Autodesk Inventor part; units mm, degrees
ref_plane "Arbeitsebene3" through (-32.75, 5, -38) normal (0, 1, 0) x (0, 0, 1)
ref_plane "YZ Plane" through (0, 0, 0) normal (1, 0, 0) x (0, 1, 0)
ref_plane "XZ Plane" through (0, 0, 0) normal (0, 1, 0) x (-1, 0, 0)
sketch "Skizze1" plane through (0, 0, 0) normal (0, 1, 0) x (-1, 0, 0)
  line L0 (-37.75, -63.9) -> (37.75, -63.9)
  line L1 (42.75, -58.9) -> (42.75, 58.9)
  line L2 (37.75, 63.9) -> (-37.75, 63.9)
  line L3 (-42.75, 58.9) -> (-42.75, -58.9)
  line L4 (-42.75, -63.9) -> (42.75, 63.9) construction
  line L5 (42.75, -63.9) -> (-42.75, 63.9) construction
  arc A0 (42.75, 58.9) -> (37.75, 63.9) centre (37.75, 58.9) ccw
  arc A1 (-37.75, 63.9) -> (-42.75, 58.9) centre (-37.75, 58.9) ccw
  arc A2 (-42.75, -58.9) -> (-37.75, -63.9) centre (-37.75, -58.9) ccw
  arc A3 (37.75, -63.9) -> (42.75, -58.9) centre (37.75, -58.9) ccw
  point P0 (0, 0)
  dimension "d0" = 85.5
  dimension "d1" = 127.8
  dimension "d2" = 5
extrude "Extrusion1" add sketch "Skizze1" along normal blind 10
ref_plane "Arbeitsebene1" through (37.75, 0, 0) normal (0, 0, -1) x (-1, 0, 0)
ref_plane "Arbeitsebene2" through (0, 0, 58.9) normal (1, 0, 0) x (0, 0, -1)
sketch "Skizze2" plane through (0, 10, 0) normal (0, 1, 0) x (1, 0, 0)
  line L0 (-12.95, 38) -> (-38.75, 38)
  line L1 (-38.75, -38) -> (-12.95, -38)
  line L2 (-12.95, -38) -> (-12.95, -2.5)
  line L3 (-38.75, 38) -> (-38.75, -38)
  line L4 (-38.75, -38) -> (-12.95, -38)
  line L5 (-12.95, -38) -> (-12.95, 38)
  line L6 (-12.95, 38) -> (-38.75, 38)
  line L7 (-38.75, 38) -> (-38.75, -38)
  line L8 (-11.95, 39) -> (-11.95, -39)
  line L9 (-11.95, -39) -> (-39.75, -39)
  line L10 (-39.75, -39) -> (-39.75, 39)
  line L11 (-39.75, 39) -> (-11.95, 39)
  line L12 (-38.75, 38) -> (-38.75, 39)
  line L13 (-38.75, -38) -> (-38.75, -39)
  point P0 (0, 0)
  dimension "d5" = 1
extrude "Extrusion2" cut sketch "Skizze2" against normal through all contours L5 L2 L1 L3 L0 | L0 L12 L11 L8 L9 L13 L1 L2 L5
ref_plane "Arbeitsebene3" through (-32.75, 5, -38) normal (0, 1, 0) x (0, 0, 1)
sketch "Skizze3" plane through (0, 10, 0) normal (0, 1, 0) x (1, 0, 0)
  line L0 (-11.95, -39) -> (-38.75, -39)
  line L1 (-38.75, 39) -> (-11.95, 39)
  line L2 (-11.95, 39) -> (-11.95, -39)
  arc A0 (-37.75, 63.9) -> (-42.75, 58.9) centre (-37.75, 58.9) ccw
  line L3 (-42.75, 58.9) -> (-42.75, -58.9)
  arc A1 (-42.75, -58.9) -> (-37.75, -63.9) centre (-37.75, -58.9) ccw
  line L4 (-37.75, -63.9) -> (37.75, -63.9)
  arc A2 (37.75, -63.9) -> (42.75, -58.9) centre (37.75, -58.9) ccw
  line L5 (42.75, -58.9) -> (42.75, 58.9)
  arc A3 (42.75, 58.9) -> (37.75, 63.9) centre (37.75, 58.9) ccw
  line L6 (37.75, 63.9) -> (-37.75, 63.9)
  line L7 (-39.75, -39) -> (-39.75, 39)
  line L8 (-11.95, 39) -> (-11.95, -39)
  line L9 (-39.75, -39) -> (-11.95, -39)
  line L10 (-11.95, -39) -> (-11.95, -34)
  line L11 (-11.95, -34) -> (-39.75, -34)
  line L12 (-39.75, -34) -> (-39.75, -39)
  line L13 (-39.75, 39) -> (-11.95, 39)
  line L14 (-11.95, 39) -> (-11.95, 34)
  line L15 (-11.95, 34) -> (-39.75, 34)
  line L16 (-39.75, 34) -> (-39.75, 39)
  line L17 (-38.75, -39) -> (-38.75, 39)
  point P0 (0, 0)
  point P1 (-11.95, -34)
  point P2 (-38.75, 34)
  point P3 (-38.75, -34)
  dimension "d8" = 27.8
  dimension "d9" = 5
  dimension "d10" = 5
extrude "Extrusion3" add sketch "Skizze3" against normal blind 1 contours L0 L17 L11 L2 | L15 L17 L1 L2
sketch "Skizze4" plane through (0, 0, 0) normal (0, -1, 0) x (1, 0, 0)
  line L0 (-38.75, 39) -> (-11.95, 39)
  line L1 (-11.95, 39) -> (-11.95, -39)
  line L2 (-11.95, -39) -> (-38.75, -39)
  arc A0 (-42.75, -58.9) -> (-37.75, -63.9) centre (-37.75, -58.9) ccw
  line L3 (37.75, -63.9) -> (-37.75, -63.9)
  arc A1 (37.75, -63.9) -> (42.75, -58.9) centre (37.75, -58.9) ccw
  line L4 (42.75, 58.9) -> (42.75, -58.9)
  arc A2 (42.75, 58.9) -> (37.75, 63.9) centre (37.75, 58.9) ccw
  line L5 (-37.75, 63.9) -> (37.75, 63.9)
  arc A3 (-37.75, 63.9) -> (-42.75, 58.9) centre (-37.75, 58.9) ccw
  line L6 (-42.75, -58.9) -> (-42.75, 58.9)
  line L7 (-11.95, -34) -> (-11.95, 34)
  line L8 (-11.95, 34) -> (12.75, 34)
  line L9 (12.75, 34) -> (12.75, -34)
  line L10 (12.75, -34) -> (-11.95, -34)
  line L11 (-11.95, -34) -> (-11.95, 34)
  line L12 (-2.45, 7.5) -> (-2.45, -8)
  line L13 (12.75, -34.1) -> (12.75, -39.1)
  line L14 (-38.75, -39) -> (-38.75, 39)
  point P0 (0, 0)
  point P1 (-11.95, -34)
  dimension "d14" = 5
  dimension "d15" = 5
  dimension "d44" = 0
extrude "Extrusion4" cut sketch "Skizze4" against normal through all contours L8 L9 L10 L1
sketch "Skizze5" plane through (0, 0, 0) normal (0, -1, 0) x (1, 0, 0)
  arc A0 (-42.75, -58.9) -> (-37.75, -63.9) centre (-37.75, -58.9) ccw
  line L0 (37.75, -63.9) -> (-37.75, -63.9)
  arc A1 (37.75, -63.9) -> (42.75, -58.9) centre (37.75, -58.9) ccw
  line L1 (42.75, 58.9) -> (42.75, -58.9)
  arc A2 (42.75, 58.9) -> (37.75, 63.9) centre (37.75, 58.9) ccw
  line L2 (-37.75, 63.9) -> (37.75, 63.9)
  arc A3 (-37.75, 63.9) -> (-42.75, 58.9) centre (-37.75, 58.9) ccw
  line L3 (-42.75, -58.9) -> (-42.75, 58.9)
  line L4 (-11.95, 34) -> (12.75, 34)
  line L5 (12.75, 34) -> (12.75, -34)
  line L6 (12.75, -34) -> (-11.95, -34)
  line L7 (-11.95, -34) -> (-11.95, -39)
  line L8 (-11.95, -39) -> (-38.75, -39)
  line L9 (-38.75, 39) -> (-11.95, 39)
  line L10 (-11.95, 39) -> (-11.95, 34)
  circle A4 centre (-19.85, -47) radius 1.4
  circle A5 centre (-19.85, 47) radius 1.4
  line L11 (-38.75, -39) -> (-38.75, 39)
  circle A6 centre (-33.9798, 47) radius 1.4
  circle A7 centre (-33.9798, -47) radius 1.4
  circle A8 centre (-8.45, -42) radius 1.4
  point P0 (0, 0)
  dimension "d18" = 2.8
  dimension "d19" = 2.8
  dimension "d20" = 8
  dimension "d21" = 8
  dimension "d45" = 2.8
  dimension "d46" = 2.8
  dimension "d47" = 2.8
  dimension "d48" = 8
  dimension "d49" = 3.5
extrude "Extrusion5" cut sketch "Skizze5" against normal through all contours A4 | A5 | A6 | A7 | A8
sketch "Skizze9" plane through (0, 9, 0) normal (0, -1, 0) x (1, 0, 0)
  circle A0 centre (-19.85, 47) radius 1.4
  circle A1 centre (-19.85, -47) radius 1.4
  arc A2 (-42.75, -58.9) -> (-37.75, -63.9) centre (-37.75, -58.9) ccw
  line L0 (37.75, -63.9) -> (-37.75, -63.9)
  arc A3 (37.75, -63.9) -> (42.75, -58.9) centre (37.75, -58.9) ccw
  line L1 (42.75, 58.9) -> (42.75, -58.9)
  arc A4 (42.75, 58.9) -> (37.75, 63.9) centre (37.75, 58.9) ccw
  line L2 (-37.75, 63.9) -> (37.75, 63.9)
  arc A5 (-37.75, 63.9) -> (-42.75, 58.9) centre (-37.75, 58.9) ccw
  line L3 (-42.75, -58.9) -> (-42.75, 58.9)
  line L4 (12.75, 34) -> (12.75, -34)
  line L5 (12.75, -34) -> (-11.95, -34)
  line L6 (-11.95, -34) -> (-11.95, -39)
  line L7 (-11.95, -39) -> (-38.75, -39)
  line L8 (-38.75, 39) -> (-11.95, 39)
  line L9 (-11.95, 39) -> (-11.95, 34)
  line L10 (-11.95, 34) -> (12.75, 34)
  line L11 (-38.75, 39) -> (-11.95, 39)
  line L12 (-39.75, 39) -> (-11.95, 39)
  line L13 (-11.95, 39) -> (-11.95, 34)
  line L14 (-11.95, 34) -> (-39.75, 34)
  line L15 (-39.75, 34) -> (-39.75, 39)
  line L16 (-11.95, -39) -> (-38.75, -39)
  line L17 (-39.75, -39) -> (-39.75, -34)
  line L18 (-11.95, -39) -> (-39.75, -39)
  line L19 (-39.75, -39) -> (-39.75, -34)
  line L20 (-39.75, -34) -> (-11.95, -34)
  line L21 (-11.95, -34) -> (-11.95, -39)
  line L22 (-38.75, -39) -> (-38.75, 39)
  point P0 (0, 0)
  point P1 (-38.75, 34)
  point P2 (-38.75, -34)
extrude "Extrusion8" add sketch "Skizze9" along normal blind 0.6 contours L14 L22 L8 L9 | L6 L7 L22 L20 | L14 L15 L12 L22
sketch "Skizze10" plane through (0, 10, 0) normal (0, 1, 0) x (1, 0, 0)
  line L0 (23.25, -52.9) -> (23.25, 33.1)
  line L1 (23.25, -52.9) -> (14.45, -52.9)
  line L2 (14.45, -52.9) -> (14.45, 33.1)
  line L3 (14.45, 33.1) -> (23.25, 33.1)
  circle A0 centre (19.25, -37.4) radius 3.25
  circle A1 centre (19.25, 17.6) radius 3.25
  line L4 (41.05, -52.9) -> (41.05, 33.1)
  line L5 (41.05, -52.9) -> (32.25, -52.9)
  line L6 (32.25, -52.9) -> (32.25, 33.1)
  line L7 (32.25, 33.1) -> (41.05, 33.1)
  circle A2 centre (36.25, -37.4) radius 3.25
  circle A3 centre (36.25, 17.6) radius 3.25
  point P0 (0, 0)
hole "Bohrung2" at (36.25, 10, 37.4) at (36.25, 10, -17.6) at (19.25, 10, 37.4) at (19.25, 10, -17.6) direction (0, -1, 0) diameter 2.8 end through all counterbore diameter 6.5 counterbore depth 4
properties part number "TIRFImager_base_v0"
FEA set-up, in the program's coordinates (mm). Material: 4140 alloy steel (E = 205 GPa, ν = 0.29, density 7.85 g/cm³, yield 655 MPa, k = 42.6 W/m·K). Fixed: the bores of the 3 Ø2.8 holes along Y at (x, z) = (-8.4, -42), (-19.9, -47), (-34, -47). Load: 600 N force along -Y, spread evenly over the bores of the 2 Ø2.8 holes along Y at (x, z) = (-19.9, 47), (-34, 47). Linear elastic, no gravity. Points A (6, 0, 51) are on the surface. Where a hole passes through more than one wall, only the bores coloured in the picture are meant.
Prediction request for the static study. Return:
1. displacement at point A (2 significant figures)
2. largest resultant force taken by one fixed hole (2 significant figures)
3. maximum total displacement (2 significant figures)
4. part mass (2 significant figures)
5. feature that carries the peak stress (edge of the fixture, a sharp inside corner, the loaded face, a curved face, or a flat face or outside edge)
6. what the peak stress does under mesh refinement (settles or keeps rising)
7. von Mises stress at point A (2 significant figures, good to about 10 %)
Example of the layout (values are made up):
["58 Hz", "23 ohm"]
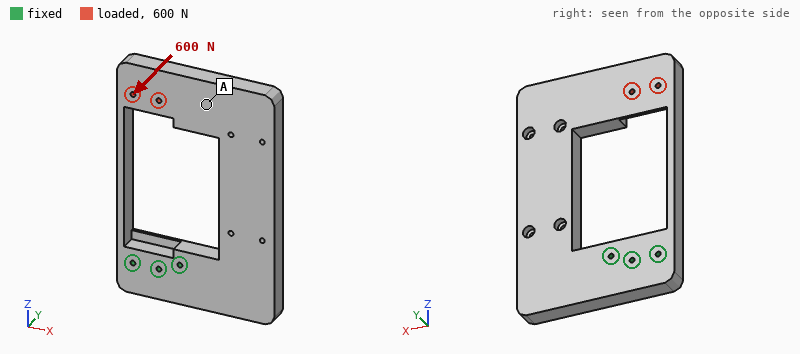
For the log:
["0.47 mm", "880 N", "0.68 mm", "560 g", "edge of the fixture", "keeps rising", "20 MPa"]
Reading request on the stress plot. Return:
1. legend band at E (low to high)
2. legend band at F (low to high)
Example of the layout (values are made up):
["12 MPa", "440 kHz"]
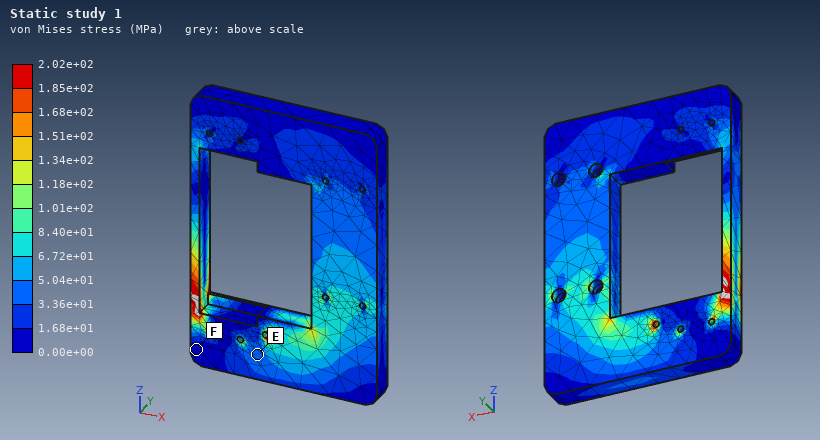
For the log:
["3.36e+01 to 5.04e+01 MPa", "0.00e+00 to 1.68e+01 MPa"]
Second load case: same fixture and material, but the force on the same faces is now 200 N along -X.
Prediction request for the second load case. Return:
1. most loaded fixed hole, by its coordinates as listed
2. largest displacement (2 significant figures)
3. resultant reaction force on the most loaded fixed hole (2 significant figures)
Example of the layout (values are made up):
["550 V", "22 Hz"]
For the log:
["(-8.4, -42)", "19 µm", "920 N"]
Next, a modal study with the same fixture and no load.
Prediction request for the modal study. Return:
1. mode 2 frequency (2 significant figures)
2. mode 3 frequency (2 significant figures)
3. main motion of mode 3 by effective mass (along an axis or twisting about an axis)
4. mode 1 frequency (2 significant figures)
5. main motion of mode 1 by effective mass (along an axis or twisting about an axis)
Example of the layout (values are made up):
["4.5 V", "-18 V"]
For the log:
["980 Hz", "1100 Hz", "along X", "370 Hz", "along Y"]
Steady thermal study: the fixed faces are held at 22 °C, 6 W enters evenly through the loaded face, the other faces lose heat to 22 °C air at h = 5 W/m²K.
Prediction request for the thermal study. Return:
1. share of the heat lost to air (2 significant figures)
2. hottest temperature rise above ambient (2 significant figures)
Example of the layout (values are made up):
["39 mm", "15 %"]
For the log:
["37 %", "48 K"]
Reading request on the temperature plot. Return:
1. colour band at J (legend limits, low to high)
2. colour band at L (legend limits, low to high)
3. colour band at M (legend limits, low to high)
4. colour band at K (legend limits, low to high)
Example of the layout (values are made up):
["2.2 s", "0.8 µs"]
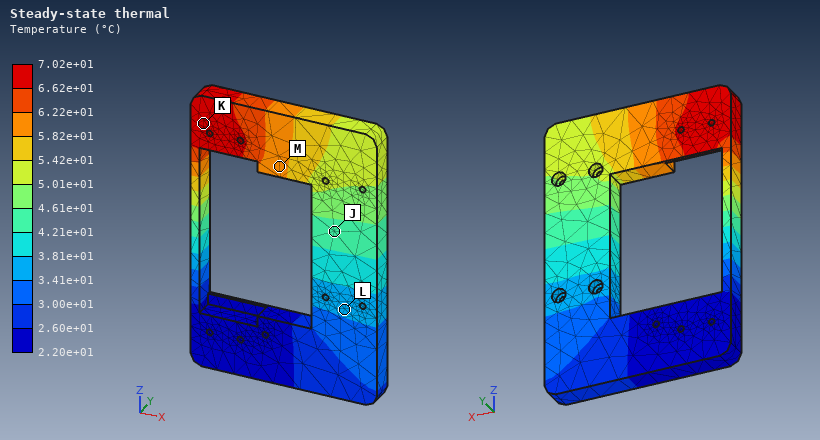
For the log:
["4.21e+01 to 4.61e+01 °C", "3.41e+01 to 3.81e+01 °C", "5.82e+01 to 6.22e+01 °C", "6.62e+01 to 7.02e+01 °C"]
